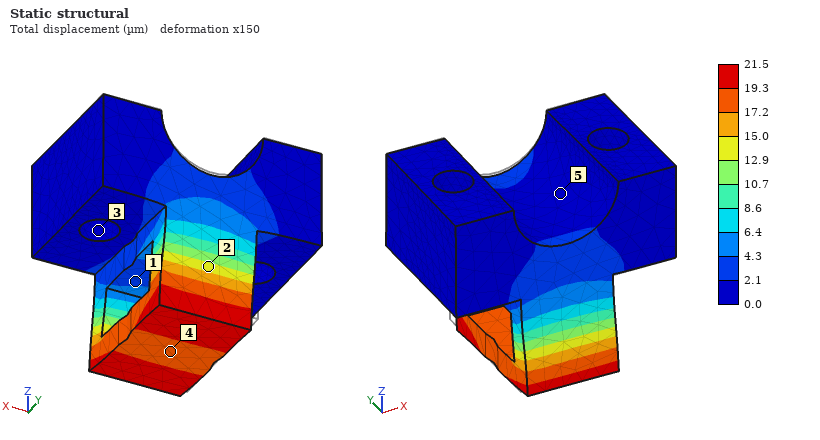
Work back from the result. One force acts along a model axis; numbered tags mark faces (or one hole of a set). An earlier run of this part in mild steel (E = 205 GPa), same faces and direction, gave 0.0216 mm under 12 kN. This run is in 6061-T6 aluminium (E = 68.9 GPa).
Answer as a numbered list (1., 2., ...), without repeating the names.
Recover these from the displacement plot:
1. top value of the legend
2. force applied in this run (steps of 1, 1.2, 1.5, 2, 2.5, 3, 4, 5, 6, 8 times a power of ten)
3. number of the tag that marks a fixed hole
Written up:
1. 21.5 µm
2. 4 kN
3. 3
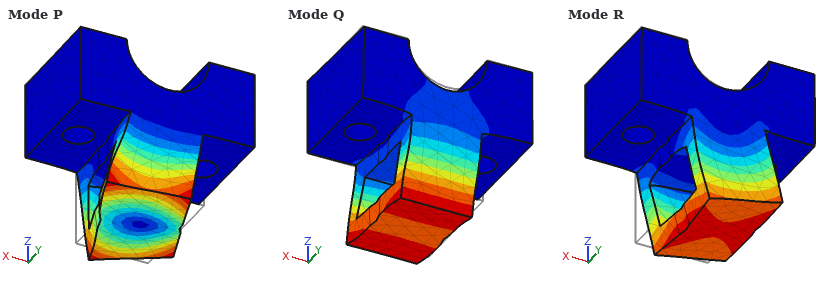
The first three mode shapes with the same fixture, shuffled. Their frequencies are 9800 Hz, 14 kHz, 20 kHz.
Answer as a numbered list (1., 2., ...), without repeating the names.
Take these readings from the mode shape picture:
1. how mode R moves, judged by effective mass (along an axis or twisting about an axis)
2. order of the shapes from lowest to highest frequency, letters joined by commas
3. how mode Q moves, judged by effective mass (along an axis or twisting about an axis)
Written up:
1. along X
2. Q, R, P
3. along Y
